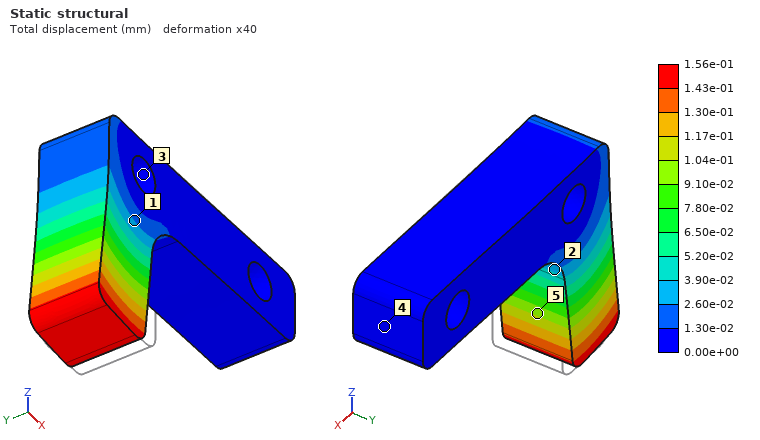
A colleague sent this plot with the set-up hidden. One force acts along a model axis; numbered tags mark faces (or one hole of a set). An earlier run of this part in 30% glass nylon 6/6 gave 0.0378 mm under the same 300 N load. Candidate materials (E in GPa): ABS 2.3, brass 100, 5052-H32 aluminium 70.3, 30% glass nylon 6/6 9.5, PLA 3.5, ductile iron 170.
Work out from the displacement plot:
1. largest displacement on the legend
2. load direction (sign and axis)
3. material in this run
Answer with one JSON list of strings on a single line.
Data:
["1.56e-01 mm", "-X", "ABS"]
